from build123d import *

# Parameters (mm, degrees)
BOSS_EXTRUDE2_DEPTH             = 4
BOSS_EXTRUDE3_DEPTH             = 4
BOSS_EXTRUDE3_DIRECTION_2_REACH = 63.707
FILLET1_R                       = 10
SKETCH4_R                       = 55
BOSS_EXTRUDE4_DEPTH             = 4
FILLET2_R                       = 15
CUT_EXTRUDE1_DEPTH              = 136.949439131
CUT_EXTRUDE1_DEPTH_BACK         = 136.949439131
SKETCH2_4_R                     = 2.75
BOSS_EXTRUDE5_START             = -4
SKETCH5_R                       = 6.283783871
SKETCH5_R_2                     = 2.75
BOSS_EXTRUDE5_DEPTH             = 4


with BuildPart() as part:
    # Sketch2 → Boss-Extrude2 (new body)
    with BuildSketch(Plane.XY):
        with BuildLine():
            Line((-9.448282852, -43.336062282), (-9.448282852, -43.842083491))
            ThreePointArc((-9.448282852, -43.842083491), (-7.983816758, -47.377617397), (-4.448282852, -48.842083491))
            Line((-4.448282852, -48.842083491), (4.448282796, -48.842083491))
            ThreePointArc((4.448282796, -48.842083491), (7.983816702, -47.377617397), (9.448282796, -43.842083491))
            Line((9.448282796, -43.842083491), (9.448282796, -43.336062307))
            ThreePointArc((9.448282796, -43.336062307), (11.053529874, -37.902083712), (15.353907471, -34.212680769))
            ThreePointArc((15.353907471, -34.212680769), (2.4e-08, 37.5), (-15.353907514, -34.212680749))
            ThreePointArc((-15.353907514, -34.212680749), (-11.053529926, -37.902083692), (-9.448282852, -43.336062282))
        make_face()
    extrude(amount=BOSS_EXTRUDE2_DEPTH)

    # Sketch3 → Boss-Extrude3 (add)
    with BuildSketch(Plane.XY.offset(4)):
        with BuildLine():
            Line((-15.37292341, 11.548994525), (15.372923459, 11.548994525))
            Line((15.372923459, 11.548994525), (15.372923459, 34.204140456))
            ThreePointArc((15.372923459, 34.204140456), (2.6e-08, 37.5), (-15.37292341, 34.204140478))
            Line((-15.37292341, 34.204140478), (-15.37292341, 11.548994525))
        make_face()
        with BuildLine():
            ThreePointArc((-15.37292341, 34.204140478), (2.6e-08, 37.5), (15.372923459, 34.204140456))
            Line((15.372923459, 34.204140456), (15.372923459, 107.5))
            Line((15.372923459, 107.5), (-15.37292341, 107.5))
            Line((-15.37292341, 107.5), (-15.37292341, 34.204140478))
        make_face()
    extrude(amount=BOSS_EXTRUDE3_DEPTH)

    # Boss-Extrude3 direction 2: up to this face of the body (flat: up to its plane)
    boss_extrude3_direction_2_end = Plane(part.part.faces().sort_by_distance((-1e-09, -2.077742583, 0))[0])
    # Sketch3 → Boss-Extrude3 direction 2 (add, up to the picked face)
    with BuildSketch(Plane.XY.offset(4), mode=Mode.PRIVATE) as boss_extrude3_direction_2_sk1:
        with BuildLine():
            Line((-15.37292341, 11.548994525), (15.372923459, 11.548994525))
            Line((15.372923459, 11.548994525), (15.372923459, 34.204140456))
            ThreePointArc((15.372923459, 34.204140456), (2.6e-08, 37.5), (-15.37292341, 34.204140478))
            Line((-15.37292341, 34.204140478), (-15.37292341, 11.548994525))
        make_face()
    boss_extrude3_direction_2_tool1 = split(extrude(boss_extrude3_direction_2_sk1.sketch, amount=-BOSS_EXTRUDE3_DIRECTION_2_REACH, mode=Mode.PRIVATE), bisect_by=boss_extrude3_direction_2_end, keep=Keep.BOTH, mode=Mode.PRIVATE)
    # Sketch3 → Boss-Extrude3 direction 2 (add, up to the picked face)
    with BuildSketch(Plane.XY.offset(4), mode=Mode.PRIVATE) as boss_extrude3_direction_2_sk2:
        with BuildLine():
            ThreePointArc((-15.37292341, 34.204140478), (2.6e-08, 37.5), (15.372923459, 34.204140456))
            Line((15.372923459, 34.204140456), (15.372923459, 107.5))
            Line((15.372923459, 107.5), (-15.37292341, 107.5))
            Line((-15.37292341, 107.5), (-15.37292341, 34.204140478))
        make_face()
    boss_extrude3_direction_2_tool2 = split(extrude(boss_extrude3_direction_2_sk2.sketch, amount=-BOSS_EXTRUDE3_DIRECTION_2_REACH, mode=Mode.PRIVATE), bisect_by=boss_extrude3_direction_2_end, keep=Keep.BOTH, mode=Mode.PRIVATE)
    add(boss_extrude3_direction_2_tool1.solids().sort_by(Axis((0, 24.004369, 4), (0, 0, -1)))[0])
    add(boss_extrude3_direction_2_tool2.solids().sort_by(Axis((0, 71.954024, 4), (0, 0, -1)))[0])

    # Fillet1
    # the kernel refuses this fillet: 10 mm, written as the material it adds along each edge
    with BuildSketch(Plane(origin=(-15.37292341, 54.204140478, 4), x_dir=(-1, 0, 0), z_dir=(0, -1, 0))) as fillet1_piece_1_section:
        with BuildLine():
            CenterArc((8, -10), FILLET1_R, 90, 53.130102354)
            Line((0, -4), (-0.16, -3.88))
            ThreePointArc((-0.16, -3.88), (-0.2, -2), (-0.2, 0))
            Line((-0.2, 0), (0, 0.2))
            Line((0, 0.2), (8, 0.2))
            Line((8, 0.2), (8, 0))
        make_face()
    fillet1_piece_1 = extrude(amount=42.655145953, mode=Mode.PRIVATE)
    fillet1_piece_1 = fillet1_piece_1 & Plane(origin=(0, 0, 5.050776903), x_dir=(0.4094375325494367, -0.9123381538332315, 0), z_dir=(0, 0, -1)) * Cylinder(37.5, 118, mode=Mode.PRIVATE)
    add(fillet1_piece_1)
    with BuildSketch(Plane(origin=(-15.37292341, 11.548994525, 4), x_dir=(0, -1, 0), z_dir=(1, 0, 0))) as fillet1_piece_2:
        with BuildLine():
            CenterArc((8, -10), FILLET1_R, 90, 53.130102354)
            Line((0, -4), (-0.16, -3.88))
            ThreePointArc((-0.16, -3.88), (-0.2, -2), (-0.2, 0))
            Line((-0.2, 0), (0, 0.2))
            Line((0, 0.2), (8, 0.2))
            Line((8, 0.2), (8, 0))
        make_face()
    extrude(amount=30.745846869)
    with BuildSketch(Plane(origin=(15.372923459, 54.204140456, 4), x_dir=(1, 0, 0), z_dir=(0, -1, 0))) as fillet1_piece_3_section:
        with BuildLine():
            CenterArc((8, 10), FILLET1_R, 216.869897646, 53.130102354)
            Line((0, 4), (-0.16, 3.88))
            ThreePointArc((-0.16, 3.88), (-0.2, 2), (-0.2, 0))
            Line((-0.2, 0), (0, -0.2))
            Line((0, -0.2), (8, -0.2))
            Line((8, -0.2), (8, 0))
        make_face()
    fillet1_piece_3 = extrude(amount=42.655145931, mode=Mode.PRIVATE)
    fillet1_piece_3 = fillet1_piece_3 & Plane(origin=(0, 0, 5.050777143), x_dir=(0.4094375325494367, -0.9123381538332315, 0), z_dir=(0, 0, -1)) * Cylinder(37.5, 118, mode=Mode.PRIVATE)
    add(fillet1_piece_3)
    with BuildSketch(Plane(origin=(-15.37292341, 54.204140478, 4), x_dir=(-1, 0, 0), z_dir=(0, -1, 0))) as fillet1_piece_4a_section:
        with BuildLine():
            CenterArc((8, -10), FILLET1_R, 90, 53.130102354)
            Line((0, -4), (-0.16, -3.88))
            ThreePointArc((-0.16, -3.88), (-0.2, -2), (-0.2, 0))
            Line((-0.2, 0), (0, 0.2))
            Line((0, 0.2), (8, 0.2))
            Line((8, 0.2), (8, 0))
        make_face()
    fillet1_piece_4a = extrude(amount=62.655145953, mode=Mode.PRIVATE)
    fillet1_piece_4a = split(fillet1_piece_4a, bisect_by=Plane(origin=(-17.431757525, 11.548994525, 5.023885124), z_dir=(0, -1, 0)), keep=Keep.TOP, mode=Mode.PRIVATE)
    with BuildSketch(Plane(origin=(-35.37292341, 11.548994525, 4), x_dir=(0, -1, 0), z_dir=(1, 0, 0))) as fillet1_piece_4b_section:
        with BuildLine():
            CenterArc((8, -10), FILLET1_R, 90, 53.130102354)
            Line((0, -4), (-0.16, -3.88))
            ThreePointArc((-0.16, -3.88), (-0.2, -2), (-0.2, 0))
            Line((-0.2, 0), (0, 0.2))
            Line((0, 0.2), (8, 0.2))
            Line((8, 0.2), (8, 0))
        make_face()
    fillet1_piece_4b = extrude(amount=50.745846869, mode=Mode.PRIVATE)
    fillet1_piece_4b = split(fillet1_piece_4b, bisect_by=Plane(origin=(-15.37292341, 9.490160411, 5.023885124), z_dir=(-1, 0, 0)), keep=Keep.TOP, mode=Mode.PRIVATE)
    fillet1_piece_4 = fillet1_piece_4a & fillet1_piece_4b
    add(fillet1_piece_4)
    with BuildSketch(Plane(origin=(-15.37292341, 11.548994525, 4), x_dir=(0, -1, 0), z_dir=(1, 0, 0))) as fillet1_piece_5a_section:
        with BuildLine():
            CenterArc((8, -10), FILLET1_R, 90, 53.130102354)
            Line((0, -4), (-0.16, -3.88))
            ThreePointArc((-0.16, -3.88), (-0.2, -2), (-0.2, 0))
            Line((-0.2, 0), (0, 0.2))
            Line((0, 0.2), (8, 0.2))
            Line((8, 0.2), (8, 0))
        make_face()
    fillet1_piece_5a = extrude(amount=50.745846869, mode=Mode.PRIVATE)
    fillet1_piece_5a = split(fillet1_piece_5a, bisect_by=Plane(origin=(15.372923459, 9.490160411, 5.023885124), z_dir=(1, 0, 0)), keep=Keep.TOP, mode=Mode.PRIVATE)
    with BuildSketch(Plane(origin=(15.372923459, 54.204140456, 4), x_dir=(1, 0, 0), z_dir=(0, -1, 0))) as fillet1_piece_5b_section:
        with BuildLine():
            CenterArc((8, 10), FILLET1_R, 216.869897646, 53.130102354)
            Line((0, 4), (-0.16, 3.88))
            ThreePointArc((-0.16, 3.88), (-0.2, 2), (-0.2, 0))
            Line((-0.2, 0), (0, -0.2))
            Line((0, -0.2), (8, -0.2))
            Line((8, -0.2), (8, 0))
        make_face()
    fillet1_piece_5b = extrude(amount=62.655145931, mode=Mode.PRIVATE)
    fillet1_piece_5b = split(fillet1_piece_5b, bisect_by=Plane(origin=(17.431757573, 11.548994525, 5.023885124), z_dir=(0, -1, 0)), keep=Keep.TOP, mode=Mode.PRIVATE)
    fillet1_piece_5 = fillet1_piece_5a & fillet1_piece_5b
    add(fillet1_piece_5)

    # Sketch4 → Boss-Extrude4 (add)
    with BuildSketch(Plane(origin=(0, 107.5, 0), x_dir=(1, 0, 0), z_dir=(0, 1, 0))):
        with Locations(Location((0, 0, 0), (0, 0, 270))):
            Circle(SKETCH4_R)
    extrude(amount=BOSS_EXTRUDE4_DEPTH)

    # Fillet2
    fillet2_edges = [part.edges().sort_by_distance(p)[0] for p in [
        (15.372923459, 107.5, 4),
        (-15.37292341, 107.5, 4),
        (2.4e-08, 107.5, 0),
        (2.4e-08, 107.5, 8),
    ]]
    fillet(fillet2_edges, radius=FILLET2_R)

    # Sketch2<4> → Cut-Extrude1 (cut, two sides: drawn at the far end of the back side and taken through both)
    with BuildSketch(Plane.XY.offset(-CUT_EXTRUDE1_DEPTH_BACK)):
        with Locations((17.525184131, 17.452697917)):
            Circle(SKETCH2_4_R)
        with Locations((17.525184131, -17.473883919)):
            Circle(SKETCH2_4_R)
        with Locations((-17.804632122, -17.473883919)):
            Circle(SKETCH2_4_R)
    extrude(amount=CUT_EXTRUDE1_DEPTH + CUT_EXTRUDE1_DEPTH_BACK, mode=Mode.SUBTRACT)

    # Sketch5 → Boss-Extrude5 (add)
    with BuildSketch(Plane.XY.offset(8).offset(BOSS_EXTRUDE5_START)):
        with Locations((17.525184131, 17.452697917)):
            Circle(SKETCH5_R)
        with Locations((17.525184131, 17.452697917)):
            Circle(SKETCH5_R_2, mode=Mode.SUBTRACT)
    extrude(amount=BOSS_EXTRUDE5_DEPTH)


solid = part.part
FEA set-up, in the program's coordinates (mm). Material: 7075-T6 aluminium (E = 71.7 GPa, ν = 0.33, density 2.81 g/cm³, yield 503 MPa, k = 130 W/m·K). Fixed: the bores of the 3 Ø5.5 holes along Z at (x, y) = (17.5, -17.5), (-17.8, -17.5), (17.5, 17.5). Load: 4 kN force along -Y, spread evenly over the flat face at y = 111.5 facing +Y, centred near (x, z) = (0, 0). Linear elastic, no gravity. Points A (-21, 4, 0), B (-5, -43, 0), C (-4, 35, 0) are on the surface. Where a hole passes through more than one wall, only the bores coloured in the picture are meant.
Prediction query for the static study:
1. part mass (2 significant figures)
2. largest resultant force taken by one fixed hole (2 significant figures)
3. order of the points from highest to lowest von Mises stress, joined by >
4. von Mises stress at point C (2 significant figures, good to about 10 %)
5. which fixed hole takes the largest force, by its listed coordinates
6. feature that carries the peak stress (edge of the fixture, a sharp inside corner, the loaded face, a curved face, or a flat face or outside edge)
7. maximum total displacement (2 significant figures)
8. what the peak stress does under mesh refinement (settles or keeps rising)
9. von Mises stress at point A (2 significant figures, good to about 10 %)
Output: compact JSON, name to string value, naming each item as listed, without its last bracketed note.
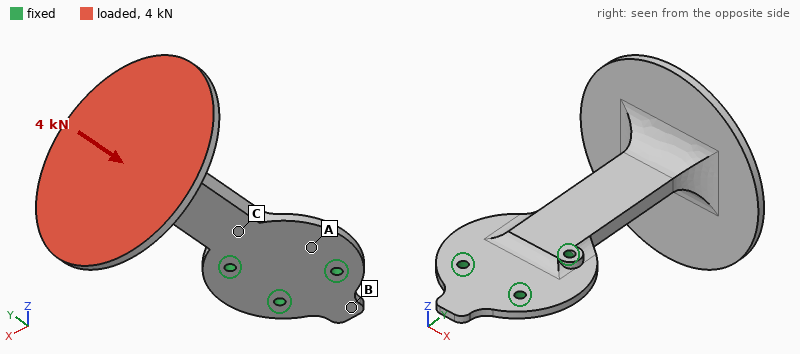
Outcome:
{"part mass": "230 g", "largest resultant force taken by one fixed hole": "1.9 kN", "order of the points from highest to lowest von Mises stress, joined by >": "C > A > B", "von Mises stress at point C": "55 MPa", "which fixed hole takes the largest force, by its listed coordinates": "(17.5, 17.5)", "feature that carries the peak stress": "edge of the fixture", "maximum total displacement": "1.5 mm", "what the peak stress does under mesh refinement": "keeps rising", "von Mises stress at point A": "24 MPa"}
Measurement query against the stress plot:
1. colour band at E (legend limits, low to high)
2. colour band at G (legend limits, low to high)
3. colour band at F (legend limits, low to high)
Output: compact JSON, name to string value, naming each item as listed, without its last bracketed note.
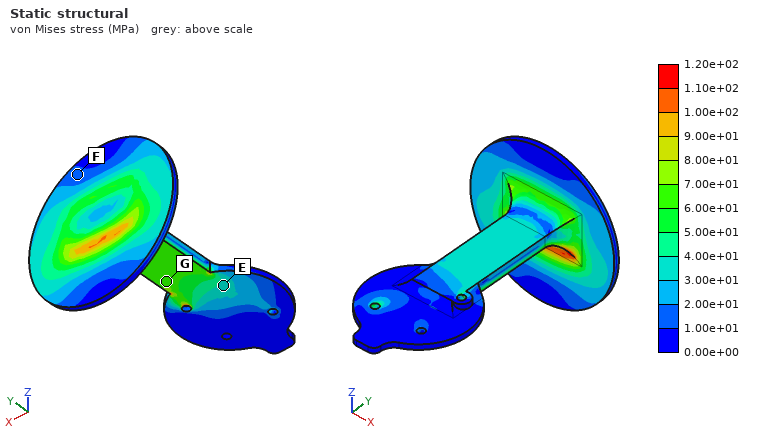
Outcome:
{"colour band at E": "3.00e+01 to 4.00e+01 MPa", "colour band at G": "6.00e+01 to 7.00e+01 MPa", "colour band at F": "1.00e+01 to 2.00e+01 MPa"}
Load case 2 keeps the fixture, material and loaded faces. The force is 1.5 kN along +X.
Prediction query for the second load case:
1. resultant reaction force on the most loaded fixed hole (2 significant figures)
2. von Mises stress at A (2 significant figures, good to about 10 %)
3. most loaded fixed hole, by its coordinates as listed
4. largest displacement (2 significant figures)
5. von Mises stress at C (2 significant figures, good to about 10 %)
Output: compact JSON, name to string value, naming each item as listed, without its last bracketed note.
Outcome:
{"resultant reaction force on the most loaded fixed hole": "3.8 kN", "von Mises stress at A": "24 MPa", "most loaded fixed hole, by its coordinates as listed": "(17.5, 17.5)", "largest displacement": "0.62 mm", "von Mises stress at C": "26 MPa"}
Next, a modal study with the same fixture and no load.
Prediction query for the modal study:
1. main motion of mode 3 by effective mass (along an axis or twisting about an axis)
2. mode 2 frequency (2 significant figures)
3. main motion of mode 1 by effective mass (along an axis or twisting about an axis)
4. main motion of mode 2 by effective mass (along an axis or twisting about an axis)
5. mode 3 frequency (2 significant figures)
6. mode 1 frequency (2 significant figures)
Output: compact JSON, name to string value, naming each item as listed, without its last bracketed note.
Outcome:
{"main motion of mode 3 by effective mass": "along X", "mode 2 frequency": "460 Hz", "main motion of mode 1 by effective mass": "along Z", "main motion of mode 2 by effective mass": "twisting about Y", "mode 3 frequency": "930 Hz", "mode 1 frequency": "230 Hz"}
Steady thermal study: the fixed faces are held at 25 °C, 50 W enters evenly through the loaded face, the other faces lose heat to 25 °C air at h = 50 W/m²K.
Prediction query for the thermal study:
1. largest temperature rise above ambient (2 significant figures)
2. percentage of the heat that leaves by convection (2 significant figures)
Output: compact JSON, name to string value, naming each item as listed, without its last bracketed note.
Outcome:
{"largest temperature rise above ambient": "54 K", "percentage of the heat that leaves by convection": "72 %"}
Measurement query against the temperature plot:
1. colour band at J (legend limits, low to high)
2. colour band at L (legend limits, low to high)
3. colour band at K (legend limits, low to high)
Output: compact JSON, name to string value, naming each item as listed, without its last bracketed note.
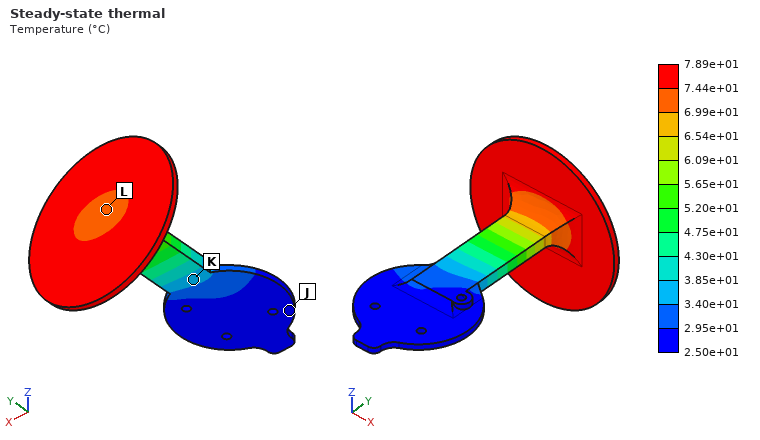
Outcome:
{"colour band at J": "2.50e+01 to 2.95e+01 °C", "colour band at L": "6.99e+01 to 7.44e+01 °C", "colour band at K": "3.40e+01 to 3.85e+01 °C"}
